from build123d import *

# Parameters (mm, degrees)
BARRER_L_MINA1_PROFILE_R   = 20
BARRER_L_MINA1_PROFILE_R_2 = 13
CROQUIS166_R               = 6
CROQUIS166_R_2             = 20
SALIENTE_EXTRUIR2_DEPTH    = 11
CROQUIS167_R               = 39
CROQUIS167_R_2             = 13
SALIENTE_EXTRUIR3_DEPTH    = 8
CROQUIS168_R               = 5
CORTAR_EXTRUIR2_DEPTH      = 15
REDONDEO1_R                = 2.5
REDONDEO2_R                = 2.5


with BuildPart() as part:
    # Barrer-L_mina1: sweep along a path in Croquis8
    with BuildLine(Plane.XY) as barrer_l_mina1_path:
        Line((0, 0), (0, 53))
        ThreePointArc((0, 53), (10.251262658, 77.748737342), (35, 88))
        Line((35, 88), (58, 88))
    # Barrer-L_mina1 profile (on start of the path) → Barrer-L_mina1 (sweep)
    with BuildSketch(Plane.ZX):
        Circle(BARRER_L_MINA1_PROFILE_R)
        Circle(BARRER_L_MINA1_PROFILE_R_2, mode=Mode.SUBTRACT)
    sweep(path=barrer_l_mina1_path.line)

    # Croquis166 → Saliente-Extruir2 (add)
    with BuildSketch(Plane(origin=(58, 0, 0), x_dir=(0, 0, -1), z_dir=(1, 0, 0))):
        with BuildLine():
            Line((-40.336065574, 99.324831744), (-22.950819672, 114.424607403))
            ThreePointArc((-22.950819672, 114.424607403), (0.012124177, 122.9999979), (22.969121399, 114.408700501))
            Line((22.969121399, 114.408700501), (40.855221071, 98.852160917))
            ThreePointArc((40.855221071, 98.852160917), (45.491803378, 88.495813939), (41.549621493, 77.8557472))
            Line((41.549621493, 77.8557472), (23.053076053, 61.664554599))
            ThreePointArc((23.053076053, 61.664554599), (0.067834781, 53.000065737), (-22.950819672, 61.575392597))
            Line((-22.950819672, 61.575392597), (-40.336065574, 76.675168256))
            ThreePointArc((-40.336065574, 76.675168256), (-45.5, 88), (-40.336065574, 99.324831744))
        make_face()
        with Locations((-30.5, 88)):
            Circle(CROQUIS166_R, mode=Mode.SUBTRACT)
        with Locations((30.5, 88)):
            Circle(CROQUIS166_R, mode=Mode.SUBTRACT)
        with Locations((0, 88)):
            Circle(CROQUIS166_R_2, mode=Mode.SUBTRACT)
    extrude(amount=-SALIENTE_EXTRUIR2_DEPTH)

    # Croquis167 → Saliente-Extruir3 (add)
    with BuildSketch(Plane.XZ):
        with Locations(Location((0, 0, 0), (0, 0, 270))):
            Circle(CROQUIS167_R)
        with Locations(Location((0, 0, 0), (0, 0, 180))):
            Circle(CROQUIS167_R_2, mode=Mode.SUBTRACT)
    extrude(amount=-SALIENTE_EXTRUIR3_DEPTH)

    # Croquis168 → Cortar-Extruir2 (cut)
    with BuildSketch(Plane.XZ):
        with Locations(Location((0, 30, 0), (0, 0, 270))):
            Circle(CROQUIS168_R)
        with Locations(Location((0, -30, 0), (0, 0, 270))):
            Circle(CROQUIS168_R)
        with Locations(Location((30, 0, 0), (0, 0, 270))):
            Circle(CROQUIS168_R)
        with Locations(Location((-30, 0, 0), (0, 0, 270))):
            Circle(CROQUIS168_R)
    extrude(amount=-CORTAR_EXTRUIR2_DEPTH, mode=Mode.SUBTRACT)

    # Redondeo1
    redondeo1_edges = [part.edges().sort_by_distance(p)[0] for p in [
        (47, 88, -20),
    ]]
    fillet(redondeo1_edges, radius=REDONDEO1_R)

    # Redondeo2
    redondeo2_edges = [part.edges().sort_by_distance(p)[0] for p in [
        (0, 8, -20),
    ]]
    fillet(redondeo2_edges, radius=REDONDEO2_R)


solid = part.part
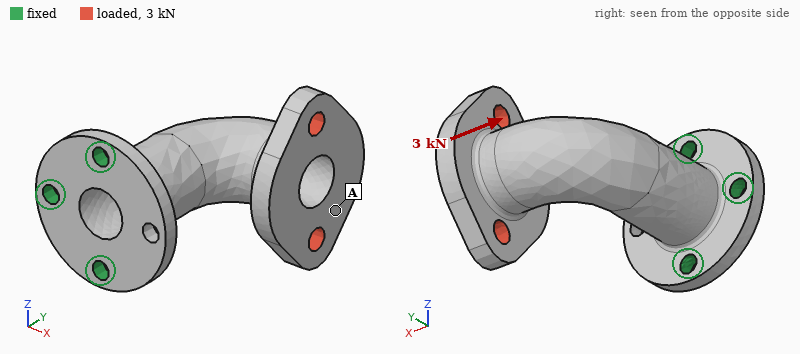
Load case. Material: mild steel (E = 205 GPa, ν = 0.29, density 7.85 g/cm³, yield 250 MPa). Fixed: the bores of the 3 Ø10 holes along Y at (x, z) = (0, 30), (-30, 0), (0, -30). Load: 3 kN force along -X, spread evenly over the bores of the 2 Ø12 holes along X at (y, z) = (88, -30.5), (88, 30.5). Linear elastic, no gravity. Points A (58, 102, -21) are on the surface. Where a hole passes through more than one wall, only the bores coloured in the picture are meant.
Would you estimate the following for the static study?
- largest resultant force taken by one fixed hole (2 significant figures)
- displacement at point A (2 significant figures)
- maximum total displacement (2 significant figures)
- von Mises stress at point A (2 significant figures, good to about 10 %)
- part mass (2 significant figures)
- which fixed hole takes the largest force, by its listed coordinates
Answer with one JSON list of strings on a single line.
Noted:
["7.6 kN", "0.15 mm", "0.17 mm", "17 MPa", "1.2 kg", "(-30, 0)"]
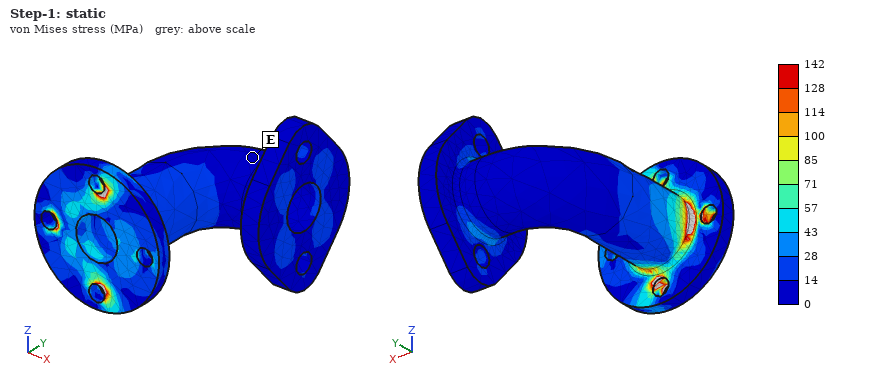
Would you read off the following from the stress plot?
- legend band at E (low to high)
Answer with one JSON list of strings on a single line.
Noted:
["0 to 14 MPa"]
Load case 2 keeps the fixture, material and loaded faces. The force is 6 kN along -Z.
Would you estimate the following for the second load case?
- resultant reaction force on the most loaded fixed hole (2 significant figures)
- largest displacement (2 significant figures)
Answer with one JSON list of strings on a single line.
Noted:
["12 kN", "0.27 mm"]
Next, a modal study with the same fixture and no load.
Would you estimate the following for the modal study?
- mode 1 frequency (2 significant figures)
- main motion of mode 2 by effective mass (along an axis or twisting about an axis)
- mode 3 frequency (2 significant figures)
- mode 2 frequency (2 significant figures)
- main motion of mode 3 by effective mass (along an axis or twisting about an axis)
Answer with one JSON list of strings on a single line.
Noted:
["890 Hz", "along Z", "3100 Hz", "1200 Hz", "twisting about Y"]
